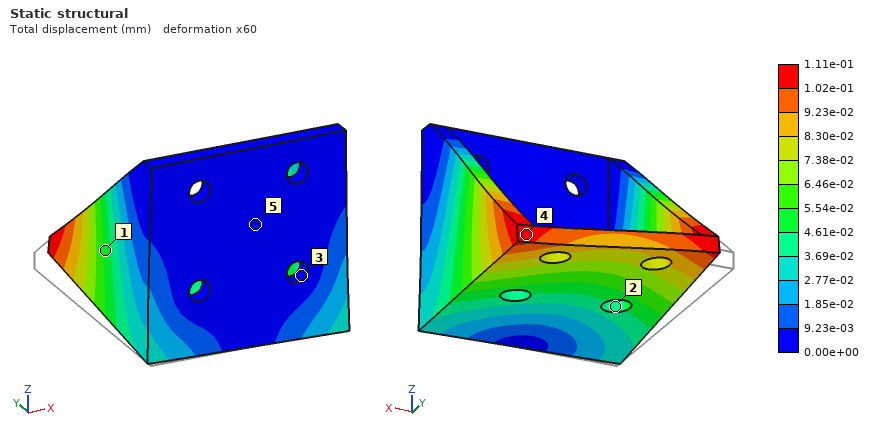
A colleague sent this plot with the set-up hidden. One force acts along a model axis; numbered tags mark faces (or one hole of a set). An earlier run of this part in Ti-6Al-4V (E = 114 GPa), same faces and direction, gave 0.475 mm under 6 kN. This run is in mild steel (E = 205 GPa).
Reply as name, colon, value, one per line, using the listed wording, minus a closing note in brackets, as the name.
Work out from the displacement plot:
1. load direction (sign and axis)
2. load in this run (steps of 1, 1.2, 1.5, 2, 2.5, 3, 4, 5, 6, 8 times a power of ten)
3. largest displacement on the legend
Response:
load direction: +X
load in this run: 2.5 kN
largest displacement on the legend: 1.11e-01 mm
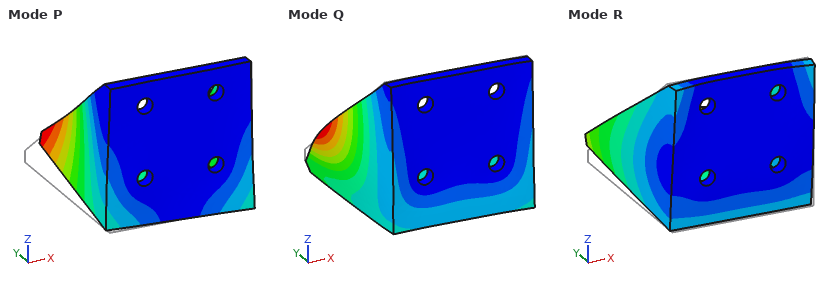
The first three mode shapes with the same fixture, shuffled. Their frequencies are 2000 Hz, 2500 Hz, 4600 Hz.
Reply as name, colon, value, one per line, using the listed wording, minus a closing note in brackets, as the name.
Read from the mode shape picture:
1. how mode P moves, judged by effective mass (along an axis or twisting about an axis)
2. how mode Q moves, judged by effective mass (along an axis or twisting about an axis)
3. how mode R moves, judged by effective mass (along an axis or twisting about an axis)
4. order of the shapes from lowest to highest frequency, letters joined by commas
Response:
how mode P moves, judged by effective mass: along X
how mode Q moves, judged by effective mass: along Y
how mode R moves, judged by effective mass: along Z
order of the shapes from lowest to highest frequency, letters joined by commas: P, R, Q
